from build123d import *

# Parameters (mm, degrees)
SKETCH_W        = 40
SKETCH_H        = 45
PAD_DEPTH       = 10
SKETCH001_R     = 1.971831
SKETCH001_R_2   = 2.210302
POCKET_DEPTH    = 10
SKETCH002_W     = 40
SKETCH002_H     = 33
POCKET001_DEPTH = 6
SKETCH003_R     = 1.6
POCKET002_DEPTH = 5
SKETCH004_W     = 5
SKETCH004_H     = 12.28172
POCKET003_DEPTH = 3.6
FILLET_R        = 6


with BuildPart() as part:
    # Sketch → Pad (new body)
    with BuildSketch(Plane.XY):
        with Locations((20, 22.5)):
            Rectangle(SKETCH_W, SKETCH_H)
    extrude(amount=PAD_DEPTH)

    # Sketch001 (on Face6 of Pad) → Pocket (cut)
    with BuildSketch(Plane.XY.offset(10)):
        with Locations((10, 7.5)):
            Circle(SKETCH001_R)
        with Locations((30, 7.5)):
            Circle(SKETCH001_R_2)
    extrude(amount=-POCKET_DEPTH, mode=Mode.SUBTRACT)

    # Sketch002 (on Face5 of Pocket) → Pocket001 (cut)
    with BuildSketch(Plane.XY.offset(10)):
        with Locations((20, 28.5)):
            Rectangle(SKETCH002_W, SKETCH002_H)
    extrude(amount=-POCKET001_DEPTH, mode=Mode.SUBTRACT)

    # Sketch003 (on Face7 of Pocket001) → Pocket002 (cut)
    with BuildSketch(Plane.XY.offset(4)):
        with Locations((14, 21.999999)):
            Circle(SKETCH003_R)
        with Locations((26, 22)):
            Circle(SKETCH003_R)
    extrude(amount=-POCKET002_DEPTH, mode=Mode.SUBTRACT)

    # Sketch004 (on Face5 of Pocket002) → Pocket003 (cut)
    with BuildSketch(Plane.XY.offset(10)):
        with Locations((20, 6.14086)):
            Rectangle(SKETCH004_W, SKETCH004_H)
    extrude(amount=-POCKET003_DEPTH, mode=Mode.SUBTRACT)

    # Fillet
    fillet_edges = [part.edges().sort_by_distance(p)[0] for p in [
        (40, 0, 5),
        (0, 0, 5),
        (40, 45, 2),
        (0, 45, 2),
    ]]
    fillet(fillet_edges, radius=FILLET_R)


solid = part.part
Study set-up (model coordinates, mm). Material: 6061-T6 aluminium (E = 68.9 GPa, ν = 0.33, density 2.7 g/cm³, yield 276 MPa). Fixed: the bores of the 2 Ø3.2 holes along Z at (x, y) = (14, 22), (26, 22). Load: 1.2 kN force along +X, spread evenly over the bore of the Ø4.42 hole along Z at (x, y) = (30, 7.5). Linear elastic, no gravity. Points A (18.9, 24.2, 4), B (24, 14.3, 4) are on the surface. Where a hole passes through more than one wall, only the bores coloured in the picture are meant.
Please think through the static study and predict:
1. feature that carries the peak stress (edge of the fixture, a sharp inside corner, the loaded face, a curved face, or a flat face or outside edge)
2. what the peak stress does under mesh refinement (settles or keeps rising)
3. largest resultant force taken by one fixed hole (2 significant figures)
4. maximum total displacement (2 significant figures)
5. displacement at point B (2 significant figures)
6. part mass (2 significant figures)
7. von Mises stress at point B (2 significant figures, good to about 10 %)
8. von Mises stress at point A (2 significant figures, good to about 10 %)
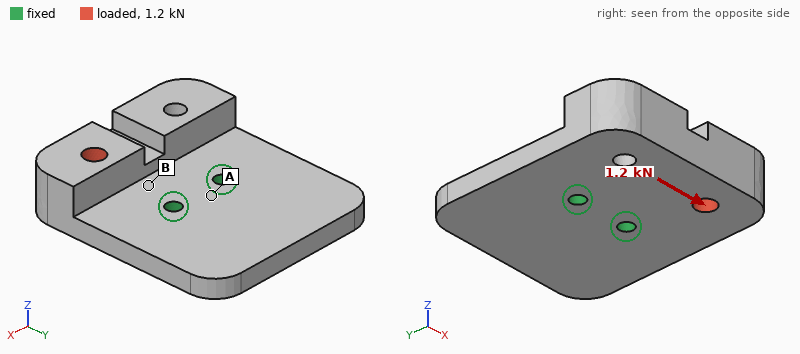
edge of the fixture
keeps rising
1.4 kN
30 µm
7.1 µm
25 g
42 MPa
8.2 MPa
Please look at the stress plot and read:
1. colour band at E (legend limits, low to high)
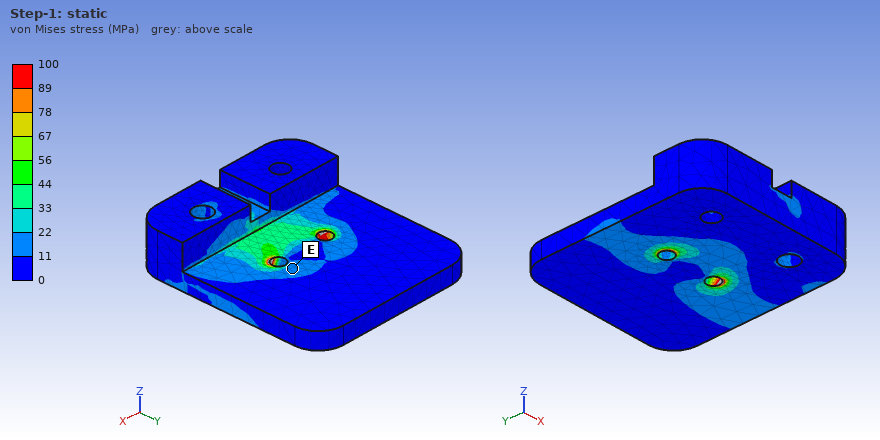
11 to 22 MPa
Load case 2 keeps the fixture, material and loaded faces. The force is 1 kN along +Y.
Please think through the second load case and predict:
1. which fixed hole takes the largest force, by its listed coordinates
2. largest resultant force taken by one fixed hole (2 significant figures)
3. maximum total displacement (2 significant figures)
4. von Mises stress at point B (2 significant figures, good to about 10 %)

(26, 22)
1.2 kN
57 µm
46 MPa
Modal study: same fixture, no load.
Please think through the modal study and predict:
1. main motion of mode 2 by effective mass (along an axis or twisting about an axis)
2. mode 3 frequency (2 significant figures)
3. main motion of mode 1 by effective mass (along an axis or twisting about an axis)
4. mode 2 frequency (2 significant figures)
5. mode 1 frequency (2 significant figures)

along Z
7100 Hz
along Z
6100 Hz
4000 Hz
